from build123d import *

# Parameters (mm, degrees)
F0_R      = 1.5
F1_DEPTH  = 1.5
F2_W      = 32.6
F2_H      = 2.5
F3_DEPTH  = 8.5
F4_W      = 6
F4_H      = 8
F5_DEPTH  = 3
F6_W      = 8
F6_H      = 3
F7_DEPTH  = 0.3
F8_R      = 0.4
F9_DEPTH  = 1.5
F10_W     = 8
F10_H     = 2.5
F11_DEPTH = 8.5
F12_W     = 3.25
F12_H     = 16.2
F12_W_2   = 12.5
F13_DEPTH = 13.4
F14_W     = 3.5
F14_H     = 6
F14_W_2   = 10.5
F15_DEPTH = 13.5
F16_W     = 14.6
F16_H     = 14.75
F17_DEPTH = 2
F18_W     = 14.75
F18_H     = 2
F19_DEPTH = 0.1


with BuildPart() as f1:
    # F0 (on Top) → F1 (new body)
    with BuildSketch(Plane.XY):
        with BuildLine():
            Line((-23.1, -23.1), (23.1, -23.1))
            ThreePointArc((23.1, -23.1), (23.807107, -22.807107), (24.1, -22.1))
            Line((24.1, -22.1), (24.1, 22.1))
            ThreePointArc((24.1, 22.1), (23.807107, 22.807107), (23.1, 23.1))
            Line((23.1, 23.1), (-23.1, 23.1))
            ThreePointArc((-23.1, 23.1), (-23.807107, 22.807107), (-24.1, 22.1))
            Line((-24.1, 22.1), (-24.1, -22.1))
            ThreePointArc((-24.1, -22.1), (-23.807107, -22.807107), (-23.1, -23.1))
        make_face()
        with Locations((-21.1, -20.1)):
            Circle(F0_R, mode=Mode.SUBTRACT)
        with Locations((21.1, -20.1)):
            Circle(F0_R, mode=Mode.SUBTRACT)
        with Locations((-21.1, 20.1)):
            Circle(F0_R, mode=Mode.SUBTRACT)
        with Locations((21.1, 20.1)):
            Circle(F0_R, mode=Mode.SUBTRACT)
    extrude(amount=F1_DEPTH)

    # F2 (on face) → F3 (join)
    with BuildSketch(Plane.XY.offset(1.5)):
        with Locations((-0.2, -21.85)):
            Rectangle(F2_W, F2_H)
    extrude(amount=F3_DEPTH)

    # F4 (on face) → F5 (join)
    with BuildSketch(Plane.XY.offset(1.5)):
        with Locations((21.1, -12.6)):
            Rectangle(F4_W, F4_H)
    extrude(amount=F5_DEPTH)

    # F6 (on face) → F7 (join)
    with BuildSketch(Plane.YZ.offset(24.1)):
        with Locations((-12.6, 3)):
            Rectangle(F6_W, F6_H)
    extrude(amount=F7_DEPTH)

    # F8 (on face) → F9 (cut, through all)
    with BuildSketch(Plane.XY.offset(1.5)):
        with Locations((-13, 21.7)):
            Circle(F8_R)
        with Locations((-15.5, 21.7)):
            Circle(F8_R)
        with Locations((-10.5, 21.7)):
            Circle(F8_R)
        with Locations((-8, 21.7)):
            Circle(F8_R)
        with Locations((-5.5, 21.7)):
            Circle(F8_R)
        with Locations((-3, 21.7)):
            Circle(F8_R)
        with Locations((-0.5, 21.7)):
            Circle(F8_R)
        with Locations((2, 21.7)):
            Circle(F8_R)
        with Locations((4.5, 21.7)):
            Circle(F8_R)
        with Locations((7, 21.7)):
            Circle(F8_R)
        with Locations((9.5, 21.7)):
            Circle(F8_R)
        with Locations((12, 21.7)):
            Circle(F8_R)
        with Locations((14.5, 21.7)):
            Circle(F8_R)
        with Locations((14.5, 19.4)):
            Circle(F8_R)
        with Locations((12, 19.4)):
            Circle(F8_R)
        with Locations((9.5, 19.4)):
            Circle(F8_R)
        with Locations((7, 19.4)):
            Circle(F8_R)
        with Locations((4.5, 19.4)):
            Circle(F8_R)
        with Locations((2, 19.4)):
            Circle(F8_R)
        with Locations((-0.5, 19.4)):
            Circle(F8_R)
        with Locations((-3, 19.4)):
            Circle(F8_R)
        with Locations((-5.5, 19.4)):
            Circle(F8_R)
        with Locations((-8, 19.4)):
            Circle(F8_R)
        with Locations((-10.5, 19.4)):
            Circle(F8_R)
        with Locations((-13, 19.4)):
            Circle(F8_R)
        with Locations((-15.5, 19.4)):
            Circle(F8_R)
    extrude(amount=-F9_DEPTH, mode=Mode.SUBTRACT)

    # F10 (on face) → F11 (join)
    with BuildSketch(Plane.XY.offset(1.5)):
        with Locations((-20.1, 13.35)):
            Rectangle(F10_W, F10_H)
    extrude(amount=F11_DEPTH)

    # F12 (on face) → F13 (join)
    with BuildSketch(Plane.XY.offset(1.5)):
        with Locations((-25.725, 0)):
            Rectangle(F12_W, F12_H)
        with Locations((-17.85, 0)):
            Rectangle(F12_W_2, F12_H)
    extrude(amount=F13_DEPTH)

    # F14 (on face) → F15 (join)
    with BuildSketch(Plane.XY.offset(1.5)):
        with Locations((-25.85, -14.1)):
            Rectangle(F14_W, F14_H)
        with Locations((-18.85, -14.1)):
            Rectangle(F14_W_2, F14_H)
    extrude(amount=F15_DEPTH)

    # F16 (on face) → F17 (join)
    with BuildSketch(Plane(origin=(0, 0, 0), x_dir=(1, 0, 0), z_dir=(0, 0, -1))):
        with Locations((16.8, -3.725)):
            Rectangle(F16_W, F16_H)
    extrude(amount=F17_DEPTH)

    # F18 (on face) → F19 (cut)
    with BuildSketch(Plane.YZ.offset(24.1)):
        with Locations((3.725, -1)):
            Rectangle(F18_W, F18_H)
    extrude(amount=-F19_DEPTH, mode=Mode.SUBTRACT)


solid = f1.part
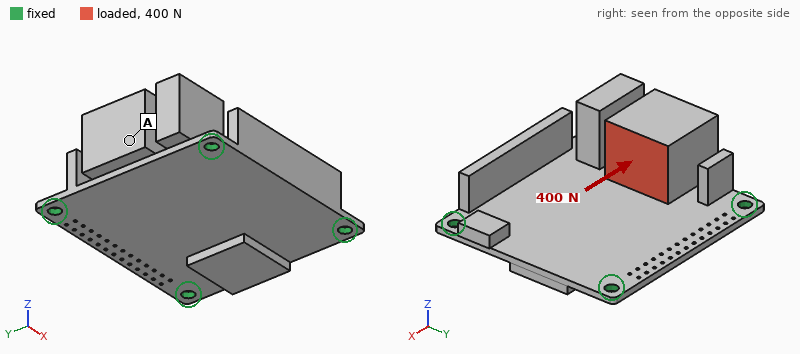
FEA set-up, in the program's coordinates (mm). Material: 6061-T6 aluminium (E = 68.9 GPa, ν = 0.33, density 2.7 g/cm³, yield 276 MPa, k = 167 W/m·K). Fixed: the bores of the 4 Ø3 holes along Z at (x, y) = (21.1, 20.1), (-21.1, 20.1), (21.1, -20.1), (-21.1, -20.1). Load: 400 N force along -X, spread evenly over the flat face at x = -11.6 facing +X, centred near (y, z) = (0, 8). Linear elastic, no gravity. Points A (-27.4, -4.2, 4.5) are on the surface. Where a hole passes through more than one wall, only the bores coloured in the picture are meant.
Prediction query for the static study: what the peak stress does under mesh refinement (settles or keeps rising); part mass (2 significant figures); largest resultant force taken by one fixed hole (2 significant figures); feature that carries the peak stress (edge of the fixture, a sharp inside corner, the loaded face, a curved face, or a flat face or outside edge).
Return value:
keeps rising
25 g
140 N
edge of the fixture
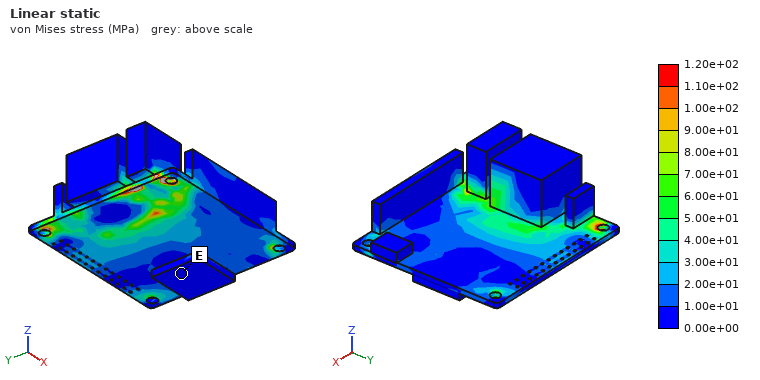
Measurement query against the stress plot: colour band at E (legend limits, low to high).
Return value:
0.00e+00 to 1.00e+01 MPa
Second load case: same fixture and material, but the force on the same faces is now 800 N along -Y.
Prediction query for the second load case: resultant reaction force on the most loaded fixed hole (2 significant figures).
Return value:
410 N
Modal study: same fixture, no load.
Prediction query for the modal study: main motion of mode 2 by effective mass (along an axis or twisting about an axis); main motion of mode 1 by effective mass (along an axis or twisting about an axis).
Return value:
along X
along Z
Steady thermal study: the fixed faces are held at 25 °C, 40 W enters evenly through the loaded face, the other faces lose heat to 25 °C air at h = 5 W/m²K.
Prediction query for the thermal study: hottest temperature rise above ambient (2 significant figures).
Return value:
66 K
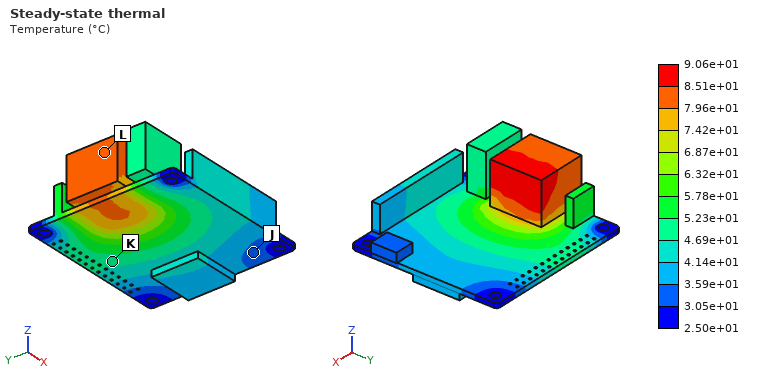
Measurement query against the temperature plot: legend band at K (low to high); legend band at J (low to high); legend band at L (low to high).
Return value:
4.69e+01 to 5.23e+01 °C
3.05e+01 to 3.59e+01 °C
7.96e+01 to 8.51e+01 °C
